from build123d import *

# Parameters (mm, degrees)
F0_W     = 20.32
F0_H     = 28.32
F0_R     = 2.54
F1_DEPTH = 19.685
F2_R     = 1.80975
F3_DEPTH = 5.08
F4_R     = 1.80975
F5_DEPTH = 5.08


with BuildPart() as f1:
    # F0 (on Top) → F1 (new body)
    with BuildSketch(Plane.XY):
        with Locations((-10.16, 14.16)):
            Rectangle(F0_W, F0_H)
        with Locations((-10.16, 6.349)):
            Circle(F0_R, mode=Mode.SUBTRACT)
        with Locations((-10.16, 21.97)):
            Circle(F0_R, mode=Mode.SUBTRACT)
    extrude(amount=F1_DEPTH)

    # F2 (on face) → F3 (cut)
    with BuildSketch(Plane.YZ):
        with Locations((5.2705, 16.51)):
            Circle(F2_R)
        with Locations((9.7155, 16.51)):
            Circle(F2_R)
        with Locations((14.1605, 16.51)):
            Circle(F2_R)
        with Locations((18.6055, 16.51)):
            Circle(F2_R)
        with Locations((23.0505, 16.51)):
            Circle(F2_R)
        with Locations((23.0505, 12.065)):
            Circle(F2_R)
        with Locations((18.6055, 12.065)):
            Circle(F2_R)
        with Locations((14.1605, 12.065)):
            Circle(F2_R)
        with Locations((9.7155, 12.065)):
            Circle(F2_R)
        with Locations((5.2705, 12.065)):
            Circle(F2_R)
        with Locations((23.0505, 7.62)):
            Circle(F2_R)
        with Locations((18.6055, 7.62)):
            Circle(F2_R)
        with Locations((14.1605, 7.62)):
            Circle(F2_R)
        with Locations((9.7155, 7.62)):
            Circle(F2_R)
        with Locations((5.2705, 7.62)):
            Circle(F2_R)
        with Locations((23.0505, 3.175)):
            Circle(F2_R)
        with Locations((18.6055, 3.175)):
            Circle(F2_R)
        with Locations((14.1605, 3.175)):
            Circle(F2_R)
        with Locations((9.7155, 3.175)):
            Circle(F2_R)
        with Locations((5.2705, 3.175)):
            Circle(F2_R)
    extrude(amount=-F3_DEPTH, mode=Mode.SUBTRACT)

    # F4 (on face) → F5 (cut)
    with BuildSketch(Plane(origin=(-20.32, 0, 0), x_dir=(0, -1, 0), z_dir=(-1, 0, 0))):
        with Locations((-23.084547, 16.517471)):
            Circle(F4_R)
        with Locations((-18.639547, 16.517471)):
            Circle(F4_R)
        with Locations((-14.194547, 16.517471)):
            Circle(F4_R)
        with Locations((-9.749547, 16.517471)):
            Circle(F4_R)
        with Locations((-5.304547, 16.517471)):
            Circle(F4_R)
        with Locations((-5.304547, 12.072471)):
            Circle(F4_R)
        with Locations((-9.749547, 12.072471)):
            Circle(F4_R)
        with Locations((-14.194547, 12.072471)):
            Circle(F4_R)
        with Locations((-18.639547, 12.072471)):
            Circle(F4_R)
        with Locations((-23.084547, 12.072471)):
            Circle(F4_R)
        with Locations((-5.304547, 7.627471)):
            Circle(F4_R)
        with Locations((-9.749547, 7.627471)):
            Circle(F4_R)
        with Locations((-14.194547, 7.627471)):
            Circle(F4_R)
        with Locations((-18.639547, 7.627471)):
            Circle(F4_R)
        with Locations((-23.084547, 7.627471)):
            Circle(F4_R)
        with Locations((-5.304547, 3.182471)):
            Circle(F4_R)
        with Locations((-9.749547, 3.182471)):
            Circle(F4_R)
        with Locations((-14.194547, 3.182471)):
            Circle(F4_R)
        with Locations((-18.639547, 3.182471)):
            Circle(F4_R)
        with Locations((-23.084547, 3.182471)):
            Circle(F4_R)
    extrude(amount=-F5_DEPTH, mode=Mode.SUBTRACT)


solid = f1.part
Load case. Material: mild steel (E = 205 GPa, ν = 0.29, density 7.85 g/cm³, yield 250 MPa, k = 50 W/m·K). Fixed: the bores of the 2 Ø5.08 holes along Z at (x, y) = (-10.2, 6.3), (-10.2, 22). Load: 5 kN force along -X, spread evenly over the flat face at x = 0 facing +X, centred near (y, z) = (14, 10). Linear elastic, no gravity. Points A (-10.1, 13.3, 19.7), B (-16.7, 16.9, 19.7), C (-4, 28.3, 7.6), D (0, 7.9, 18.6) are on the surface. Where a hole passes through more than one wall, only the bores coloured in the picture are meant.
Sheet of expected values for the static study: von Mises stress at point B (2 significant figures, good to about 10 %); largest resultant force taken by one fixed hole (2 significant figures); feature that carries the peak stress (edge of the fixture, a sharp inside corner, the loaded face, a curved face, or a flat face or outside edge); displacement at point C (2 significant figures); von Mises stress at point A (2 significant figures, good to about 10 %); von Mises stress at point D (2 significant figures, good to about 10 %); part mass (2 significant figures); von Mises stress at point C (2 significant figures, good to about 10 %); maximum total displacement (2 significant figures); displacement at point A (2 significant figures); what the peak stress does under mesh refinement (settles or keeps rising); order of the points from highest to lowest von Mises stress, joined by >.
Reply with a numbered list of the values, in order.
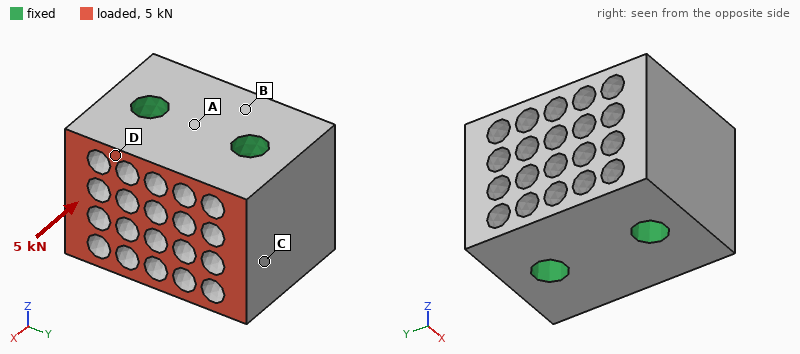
1. 2.0 MPa
2. 2.5 kN
3. edge of the fixture
4. 0.62 µm
5. 4.7 MPa
6. 16 MPa
7. 66 g
8. 12 MPa
9. 0.98 µm
10. 0.19 µm
11. keeps rising
12. D > C > A > B
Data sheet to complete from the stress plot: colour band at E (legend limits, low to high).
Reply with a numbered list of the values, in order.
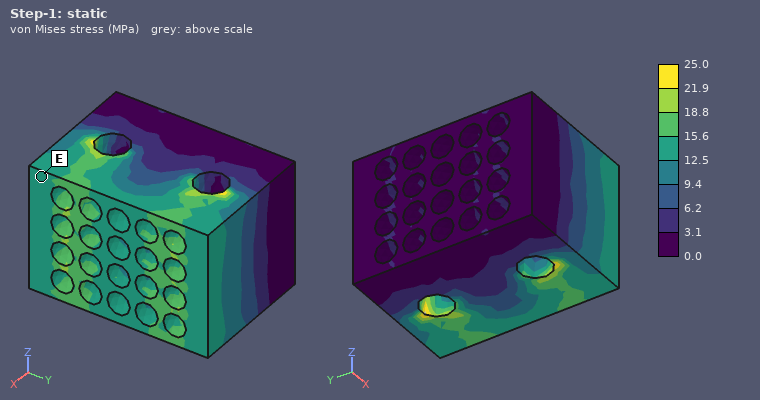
1. 12.5 to 15.6 MPa
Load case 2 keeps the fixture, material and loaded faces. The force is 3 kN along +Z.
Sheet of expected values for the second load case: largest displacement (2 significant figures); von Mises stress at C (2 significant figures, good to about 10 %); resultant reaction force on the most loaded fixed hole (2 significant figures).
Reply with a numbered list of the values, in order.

1. 2.4 µm
2. 19 MPa
3. 1.5 kN
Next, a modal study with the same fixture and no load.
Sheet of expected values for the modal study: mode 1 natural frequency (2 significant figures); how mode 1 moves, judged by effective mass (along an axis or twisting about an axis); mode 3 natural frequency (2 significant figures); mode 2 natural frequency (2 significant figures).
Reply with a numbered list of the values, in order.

1. 65 kHz
2. twisting about Z
3. 71 kHz
4. 71 kHz
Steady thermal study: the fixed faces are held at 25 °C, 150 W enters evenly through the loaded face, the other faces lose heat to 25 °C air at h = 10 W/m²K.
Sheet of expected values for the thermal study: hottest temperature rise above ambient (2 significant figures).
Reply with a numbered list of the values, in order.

1. 70 K
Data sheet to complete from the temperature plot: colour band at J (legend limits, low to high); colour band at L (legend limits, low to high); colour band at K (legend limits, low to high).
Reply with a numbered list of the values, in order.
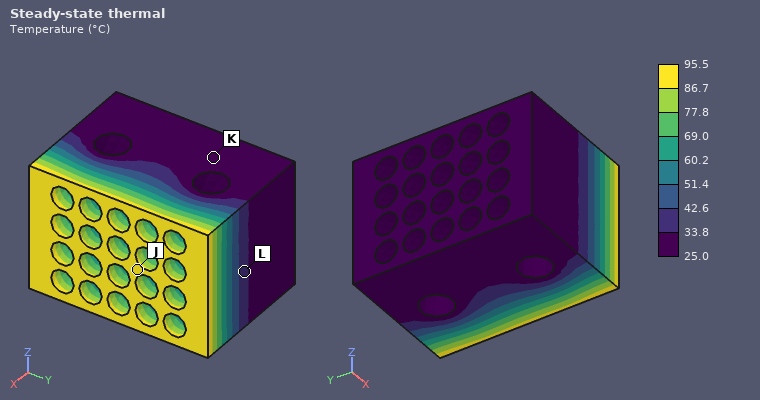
1. 86.7 to 95.5 °C
2. 33.8 to 42.6 °C
3. 25.0 to 33.8 °C
